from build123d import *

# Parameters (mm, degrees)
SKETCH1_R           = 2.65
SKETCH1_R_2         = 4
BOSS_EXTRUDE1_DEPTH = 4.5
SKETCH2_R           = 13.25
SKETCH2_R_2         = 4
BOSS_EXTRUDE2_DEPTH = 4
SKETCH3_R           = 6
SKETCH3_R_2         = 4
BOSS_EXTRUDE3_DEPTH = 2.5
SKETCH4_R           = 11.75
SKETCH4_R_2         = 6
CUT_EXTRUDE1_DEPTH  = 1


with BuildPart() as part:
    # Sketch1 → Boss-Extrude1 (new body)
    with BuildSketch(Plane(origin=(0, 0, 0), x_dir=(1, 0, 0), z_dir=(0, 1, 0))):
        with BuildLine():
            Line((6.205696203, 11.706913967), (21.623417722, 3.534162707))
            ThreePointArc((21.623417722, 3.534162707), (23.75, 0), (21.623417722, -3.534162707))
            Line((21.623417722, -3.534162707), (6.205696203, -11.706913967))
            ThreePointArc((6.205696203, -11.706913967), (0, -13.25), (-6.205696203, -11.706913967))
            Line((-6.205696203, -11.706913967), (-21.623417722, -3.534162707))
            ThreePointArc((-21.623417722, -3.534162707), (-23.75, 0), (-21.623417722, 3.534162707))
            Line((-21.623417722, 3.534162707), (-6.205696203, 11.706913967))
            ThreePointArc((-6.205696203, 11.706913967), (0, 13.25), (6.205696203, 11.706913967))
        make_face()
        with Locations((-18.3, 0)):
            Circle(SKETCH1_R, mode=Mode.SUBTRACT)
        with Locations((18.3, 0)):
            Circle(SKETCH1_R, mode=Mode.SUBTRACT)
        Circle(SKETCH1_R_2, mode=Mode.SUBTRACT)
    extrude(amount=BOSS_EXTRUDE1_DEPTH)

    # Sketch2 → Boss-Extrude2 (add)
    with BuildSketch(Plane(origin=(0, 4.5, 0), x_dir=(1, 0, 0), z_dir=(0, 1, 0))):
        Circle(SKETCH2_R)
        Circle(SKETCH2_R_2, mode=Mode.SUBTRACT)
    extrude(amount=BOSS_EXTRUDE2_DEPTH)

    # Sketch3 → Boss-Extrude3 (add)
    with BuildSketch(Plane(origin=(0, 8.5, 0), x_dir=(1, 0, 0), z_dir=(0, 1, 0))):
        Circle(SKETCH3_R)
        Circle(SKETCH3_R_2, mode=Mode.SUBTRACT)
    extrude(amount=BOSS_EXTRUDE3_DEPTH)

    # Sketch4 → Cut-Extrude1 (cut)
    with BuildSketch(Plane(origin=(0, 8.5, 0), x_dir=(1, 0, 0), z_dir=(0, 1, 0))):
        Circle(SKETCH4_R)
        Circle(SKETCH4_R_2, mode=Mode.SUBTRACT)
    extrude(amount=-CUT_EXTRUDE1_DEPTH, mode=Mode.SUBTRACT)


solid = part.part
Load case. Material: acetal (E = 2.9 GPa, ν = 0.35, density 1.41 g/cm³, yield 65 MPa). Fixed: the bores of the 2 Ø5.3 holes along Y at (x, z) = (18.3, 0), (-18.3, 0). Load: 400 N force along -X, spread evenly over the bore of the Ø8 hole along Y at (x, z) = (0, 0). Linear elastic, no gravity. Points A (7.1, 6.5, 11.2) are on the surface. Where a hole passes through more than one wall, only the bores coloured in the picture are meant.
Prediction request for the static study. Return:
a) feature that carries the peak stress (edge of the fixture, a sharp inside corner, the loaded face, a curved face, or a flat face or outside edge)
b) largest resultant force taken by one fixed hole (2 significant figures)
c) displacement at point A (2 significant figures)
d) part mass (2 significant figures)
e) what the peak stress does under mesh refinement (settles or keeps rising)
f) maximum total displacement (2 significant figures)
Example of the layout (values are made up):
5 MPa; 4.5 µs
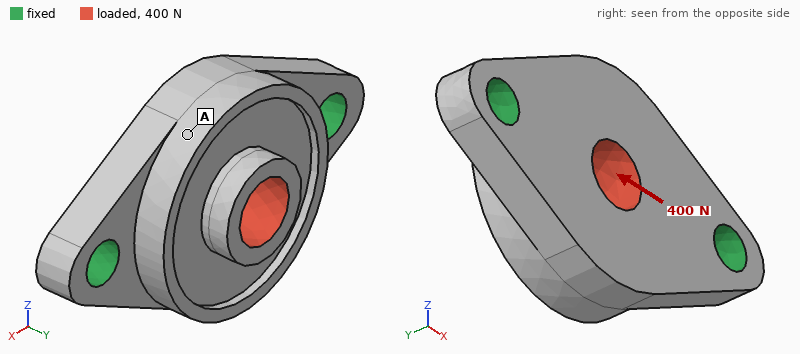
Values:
edge of the fixture; 200 N; 12 µm; 7.1 g; keeps rising; 30 µm
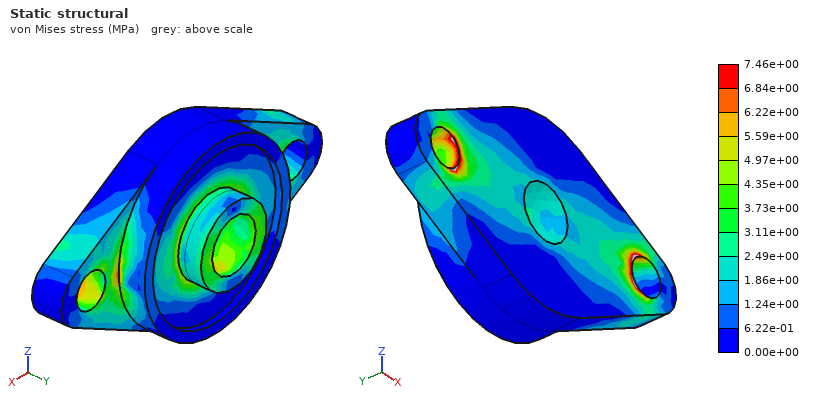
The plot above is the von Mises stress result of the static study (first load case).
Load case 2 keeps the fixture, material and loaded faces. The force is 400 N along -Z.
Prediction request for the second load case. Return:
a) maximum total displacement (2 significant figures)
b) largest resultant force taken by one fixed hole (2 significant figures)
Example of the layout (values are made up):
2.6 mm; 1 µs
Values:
0.14 mm; 200 N
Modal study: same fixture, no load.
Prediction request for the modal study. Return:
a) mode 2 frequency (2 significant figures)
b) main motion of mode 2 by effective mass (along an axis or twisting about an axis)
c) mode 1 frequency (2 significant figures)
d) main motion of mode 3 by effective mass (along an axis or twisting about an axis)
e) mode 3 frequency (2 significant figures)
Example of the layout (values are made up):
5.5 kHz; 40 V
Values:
4600 Hz; along Y; 3400 Hz; along Z; 7900 Hz
